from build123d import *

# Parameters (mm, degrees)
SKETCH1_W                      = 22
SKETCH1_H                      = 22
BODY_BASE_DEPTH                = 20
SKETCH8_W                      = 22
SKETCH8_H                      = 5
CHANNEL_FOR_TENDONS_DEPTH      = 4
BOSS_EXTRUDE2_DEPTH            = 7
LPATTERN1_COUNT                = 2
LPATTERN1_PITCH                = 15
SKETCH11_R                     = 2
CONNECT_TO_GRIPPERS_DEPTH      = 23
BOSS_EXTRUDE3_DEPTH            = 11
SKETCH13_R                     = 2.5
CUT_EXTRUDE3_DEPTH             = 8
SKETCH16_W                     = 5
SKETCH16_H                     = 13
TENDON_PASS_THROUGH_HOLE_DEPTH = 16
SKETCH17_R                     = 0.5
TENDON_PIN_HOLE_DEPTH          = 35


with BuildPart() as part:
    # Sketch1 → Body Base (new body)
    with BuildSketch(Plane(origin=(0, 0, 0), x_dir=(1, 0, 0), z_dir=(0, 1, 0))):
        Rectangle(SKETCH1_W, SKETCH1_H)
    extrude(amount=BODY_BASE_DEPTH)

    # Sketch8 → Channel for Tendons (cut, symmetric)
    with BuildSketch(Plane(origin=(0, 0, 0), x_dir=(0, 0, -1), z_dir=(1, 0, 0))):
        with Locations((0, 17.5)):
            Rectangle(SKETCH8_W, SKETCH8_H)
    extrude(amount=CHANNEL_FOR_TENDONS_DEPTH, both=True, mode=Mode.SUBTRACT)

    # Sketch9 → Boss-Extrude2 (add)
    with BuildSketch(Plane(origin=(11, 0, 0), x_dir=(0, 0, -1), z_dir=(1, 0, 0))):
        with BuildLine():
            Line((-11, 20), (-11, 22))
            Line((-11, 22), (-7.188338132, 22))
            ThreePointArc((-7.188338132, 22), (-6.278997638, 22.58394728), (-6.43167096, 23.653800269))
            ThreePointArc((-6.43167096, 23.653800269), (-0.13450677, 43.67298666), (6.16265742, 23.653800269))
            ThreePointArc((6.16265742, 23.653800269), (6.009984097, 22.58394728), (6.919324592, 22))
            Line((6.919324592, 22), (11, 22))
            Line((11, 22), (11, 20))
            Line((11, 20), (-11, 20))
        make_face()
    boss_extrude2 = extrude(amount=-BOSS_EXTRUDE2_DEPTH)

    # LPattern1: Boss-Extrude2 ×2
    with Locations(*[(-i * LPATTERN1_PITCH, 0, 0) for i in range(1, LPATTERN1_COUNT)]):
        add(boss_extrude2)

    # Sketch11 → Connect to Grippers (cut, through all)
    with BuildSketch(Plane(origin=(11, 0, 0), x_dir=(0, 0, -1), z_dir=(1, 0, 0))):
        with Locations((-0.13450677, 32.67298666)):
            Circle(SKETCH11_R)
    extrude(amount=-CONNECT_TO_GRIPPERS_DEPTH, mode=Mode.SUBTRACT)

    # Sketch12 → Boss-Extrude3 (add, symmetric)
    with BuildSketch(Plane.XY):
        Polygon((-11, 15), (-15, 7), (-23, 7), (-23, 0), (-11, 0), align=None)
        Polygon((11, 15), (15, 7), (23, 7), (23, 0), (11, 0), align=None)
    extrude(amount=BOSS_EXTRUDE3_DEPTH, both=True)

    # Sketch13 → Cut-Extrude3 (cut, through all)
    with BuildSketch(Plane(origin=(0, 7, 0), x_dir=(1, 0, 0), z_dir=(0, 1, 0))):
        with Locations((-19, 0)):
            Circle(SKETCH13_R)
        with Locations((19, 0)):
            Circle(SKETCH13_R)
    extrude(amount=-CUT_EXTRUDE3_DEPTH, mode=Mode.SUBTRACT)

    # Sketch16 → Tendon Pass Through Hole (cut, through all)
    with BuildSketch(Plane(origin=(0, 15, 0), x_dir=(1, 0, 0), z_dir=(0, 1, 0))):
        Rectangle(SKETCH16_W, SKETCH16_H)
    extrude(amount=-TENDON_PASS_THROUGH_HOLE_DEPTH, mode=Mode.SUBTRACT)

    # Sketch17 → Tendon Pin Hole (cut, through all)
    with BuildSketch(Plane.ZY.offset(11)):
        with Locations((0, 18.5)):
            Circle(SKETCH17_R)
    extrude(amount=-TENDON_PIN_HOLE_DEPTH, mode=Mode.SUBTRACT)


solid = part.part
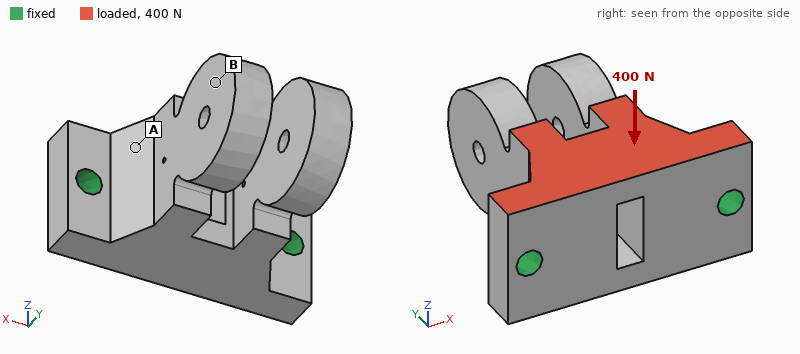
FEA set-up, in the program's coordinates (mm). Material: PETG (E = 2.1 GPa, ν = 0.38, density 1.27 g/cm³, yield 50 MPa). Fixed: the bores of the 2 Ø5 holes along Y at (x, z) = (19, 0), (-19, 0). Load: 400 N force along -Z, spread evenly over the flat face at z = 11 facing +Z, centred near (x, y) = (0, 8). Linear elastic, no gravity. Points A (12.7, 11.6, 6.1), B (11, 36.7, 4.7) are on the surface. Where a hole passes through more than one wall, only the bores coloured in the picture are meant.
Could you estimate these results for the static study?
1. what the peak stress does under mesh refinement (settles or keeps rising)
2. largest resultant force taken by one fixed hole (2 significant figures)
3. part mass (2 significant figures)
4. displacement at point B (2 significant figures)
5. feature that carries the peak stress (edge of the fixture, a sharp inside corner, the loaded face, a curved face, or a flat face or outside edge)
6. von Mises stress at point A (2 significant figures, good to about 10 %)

keeps rising
200 N
23 g
0.16 mm
edge of the fixture
2.1 MPa
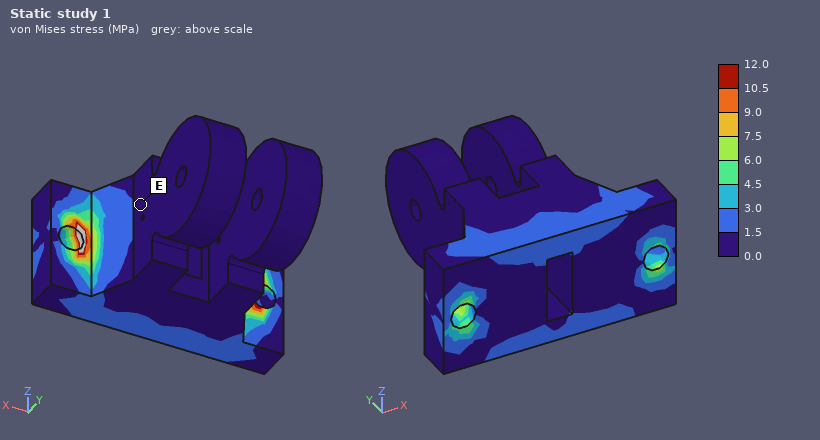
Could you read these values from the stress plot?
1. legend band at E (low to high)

0.0 to 1.5 MPa
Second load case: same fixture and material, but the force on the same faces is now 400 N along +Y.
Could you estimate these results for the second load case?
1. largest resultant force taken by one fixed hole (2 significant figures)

220 N
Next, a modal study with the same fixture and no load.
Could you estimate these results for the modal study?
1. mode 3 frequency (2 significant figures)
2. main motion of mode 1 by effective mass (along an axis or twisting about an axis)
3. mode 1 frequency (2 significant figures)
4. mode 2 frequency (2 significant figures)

1400 Hz
along Z
1200 Hz
1300 Hz
